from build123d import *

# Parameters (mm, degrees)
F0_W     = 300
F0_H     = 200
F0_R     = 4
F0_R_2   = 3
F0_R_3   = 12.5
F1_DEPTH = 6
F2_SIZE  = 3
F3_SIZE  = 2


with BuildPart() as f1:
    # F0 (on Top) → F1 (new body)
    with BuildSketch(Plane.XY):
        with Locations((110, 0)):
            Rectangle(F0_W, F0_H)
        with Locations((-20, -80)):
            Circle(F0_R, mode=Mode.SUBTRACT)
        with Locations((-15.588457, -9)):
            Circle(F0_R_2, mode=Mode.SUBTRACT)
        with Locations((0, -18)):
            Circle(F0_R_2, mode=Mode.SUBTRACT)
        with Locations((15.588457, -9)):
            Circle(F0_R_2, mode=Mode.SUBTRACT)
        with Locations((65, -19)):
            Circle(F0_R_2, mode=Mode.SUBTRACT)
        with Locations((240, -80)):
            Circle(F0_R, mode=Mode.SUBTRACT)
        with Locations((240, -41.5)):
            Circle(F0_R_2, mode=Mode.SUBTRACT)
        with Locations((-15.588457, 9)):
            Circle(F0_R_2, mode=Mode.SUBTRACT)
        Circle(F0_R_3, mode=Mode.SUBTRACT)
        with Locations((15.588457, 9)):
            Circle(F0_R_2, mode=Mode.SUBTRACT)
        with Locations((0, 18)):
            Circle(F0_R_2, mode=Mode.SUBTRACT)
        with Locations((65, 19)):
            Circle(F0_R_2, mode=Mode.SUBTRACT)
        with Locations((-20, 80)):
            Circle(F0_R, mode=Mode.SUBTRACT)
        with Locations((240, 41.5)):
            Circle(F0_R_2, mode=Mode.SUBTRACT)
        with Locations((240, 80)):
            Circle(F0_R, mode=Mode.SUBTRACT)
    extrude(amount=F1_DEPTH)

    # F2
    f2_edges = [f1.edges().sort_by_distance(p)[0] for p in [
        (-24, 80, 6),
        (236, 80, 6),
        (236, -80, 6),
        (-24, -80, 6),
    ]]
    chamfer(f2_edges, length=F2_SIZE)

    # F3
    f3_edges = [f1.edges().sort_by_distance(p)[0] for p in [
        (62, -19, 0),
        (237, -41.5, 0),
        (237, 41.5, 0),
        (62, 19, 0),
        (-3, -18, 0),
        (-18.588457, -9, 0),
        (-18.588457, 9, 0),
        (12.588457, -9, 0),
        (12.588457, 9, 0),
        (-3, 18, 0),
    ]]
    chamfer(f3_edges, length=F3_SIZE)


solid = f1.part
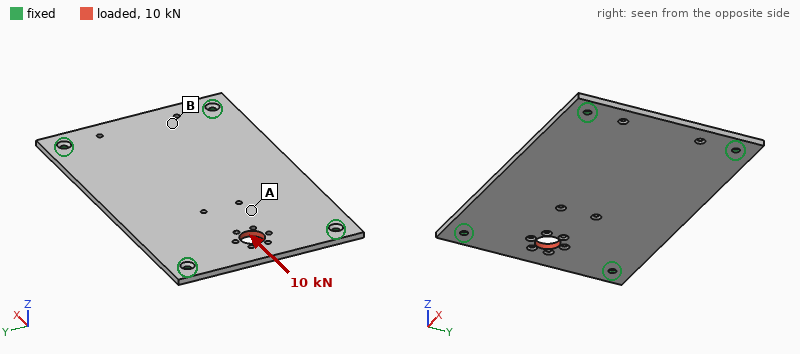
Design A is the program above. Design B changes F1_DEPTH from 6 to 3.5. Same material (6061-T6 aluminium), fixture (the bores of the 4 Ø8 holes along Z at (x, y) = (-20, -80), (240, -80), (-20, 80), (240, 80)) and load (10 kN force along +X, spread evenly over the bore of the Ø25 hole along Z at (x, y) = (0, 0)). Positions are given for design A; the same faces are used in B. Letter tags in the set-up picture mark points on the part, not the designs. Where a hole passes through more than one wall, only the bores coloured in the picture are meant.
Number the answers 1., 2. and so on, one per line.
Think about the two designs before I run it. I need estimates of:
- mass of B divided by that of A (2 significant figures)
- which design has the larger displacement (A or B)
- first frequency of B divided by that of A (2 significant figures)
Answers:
1. 0.58
2. B
3. 0.57
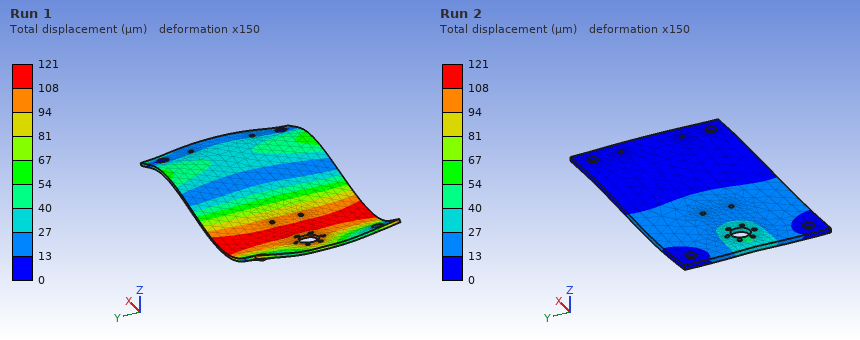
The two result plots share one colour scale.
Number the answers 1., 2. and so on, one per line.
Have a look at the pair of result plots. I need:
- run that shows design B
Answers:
1. Run 1
